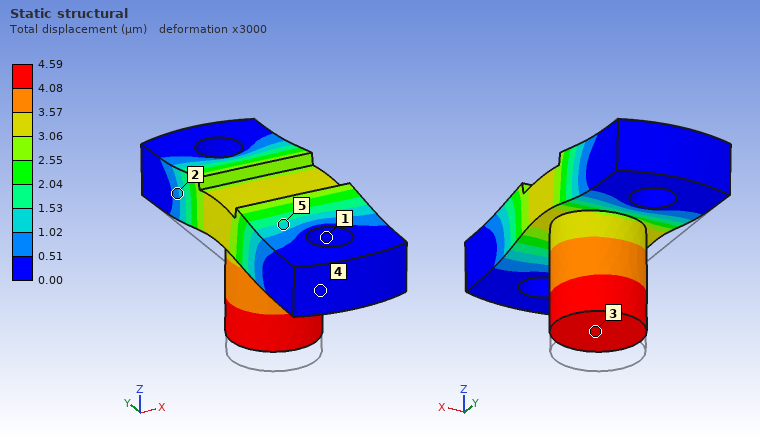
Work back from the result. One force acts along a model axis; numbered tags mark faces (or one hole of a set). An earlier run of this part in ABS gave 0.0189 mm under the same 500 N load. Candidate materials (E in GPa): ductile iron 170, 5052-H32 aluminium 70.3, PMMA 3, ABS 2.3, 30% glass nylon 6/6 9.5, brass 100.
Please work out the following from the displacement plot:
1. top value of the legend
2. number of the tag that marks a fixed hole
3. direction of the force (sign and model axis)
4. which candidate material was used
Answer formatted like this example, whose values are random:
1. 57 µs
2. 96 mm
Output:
1. 4.59 µm
2. 1
3. +Z
4. 30% glass nylon 6/6
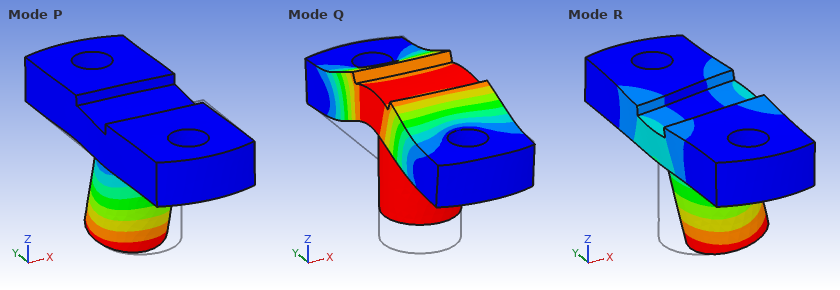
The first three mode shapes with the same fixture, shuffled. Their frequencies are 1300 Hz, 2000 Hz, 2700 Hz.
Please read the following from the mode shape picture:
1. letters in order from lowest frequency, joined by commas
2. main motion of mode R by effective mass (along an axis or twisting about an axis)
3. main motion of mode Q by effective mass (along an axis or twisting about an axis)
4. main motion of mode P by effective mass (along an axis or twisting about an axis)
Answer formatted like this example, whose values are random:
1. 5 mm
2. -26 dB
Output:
1. R, P, Q
2. along X
3. along Z
4. along Y
